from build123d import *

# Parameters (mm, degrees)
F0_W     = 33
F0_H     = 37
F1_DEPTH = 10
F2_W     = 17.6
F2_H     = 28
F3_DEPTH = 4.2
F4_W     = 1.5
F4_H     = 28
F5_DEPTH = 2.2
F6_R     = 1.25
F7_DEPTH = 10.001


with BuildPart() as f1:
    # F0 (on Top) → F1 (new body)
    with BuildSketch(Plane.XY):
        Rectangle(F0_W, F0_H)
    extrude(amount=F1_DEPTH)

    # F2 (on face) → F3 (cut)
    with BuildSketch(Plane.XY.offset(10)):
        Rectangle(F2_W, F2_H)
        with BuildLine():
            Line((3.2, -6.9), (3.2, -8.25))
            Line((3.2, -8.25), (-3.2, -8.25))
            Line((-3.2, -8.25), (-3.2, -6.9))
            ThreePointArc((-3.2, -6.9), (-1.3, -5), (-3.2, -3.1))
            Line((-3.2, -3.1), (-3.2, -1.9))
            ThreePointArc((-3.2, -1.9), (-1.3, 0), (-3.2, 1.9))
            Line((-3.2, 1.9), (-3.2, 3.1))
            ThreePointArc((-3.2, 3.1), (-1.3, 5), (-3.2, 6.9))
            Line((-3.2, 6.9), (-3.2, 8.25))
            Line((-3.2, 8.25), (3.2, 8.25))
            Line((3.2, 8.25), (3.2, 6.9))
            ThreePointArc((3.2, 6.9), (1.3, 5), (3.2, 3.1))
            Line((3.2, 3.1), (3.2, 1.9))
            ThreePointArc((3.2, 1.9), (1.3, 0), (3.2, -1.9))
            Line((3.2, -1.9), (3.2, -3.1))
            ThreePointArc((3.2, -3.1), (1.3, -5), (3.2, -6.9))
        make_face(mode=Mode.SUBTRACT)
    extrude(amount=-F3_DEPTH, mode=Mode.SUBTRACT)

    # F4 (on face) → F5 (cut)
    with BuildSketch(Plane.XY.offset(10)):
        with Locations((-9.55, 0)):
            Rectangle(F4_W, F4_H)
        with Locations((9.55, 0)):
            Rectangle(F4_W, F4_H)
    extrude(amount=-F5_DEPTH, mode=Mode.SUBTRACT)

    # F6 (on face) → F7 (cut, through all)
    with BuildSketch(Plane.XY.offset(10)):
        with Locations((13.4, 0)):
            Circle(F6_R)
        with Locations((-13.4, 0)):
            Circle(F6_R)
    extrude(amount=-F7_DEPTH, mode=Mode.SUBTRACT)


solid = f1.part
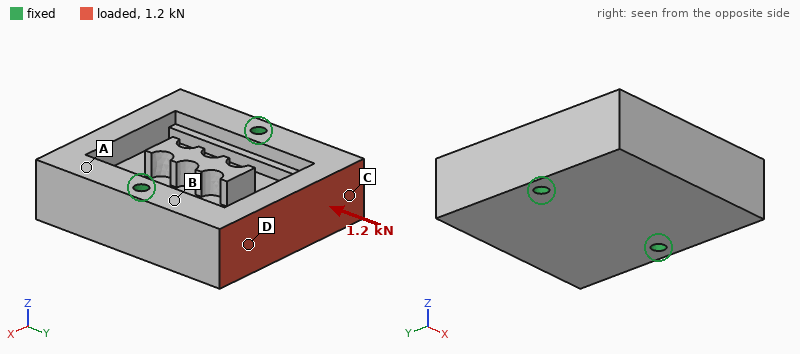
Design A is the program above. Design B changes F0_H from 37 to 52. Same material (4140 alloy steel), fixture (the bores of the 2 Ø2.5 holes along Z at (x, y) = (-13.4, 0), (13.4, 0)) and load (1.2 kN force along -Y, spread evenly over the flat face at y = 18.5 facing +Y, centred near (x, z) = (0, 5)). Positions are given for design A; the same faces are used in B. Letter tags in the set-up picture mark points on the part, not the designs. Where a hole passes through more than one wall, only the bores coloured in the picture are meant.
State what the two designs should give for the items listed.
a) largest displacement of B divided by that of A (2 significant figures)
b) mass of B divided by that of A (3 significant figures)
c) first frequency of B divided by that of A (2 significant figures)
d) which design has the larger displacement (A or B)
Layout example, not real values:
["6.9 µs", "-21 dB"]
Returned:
["0.82", "1.49", "0.55", "A"]
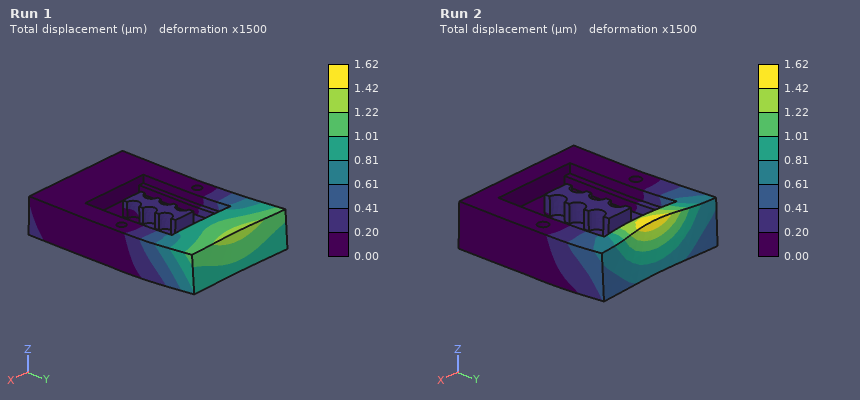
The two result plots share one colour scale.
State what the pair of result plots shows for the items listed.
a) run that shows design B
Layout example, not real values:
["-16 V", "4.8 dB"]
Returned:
["Run 1"]
